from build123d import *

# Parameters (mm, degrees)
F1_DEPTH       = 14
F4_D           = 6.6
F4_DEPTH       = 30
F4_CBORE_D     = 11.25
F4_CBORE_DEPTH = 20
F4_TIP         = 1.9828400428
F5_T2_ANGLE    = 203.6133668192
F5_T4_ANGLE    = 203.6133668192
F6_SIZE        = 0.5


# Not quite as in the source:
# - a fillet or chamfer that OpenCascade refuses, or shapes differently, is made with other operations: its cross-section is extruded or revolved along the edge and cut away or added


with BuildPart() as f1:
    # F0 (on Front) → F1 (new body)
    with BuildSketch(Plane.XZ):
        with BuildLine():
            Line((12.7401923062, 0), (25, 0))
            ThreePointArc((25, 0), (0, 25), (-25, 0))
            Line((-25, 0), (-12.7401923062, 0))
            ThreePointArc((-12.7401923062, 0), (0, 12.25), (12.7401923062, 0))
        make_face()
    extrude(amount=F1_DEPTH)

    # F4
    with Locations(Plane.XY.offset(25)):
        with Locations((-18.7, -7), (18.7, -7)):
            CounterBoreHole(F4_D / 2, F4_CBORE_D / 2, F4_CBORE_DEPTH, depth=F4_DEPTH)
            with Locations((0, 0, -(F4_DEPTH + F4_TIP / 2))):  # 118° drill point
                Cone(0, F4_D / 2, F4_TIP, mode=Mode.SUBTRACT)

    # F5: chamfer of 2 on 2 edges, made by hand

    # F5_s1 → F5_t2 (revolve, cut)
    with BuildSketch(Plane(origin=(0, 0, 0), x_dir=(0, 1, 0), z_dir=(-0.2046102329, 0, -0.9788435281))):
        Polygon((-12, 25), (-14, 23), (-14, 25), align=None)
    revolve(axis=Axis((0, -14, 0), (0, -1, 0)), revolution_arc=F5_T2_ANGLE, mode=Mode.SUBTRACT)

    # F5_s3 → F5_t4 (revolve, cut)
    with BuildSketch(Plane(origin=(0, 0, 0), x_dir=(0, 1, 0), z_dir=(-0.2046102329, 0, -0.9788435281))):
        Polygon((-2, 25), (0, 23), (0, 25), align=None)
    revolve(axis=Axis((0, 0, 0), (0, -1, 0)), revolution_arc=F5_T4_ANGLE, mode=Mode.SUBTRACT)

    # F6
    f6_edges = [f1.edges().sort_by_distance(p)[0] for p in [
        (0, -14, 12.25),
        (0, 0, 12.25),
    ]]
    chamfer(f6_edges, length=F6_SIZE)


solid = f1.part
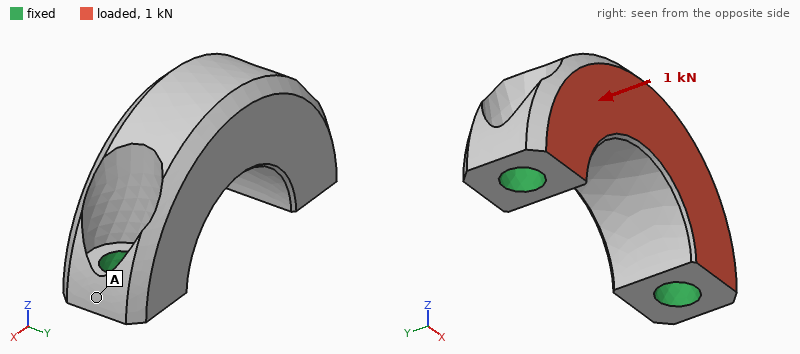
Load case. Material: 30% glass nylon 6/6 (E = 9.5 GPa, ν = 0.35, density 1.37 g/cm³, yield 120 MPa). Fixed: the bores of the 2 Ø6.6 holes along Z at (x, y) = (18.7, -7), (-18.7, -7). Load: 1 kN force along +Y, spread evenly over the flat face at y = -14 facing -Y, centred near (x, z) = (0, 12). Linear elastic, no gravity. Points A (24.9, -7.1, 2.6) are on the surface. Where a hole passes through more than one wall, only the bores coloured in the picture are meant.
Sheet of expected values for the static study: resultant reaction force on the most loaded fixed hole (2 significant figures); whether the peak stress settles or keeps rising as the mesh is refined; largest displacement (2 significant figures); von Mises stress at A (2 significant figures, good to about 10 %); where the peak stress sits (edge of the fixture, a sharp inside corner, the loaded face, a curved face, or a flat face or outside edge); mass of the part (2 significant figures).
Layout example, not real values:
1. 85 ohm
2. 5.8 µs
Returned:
1. 500 N
2. keeps rising
3. 0.15 mm
4. 8.3 MPa
5. edge of the fixture
6. 10 g
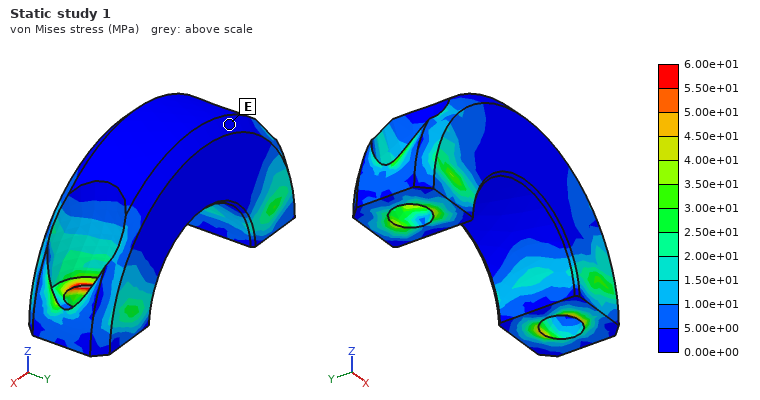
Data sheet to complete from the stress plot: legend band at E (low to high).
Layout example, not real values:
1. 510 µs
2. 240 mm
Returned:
1. 0.00e+00 to 5.00e+00 MPa
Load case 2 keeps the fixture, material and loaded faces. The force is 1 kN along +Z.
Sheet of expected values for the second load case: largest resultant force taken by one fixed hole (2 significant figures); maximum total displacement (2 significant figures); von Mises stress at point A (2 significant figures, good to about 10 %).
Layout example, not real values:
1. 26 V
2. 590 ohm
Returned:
1. 520 N
2. 94 µm
3. 4.9 MPa
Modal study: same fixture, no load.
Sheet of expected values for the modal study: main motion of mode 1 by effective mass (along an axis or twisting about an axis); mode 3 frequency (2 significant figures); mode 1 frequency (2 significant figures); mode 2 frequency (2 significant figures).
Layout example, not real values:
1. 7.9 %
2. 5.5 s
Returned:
1. along Y
2. 10 kHz
3. 4500 Hz
4. 10 kHz
